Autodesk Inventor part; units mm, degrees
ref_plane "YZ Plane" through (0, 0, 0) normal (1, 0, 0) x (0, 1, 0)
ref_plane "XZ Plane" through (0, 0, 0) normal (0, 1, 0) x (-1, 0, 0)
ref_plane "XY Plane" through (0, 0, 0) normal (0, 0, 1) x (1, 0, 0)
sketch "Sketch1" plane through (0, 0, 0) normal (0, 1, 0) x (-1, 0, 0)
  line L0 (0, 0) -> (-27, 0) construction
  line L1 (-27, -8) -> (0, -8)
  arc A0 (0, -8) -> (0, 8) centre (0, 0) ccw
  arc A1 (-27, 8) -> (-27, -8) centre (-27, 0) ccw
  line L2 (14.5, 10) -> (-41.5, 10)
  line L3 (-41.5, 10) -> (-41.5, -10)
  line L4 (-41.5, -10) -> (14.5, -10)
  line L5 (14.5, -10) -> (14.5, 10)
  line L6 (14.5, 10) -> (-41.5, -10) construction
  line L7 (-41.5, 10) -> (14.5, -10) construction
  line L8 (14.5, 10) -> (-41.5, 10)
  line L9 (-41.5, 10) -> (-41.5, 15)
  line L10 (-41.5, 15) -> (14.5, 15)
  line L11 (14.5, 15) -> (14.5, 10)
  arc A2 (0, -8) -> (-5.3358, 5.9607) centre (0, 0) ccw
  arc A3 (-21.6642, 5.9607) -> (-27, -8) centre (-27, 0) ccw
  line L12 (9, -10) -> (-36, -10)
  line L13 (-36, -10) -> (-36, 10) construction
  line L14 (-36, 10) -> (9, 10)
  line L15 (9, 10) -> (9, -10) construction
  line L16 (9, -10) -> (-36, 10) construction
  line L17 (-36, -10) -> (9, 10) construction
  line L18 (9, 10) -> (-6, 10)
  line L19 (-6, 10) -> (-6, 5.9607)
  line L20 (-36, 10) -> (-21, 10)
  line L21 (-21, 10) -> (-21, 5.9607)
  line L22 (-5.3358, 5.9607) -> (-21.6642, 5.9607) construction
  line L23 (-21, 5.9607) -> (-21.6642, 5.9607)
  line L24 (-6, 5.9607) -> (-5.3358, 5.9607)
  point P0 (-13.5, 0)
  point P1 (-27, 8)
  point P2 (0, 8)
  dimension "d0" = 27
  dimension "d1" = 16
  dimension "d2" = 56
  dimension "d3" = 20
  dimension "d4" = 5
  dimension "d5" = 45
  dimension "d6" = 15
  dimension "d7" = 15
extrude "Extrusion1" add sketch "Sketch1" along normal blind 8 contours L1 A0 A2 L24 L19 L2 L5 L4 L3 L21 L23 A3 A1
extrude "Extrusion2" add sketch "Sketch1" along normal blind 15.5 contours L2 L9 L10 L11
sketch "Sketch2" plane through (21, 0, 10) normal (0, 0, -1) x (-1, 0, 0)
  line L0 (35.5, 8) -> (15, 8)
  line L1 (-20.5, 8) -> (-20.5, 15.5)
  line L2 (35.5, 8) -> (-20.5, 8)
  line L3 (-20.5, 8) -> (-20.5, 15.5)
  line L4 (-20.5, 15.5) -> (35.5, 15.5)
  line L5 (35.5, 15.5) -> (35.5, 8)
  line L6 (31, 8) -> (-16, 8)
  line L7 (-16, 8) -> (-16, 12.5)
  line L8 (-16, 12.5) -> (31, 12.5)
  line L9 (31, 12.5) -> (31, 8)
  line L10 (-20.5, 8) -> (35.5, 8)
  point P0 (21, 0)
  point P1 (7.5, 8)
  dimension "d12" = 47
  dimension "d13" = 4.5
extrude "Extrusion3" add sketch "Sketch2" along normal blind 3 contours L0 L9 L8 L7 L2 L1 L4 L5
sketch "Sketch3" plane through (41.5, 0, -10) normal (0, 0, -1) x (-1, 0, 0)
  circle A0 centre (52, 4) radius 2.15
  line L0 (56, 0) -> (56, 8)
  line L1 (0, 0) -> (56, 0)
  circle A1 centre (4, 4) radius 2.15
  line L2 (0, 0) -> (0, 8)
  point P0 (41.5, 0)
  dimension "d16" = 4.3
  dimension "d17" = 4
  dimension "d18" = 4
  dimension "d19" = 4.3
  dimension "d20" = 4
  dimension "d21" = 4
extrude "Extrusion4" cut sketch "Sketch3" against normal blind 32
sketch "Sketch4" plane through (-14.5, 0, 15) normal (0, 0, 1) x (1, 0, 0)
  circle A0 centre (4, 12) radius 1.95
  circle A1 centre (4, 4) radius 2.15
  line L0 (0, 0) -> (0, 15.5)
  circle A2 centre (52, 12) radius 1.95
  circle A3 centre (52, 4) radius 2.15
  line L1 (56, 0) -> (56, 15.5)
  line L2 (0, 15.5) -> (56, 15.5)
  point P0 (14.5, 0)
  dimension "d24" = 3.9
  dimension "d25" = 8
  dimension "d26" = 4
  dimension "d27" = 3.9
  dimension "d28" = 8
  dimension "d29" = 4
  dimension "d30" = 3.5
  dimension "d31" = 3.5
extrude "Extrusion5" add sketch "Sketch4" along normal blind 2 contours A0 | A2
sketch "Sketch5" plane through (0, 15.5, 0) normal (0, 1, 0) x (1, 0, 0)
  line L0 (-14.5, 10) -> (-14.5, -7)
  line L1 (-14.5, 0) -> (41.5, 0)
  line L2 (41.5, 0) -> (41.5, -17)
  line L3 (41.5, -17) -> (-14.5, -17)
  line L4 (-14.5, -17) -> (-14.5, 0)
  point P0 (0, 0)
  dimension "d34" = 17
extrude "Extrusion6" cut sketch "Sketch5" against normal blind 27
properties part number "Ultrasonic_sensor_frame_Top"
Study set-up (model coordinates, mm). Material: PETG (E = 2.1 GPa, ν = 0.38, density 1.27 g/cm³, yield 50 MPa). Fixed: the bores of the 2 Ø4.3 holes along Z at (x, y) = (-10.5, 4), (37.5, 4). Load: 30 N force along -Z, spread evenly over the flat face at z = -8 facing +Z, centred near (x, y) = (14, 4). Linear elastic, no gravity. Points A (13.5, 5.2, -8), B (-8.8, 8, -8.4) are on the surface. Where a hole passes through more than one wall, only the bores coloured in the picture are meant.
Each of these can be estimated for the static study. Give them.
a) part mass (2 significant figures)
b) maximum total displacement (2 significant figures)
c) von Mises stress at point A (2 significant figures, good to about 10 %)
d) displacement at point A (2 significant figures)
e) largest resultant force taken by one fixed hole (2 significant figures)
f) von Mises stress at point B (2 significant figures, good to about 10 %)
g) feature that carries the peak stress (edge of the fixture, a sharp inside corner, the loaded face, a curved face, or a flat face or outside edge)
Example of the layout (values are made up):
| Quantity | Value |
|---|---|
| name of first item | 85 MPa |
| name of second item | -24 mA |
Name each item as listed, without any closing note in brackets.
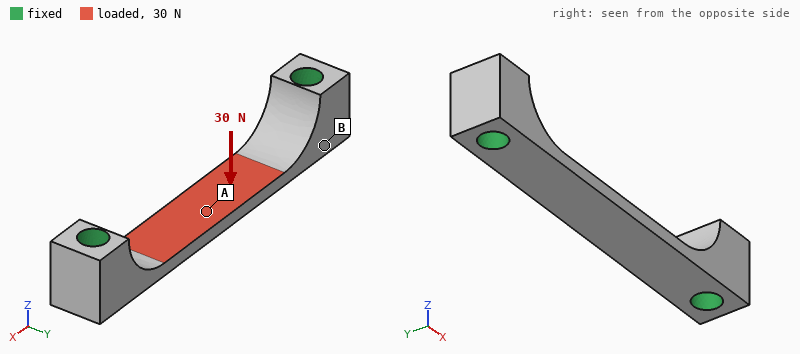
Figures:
| Quantity | Value |
|---|---|
| part mass | 2.1 g |
| maximum total displacement | 0.38 mm |
| von Mises stress at point A | 8.7 MPa |
| displacement at point A | 0.37 mm |
| largest resultant force taken by one fixed hole | 21 N |
| von Mises stress at point B | 1.6 MPa |
| feature that carries the peak stress | a curved face |
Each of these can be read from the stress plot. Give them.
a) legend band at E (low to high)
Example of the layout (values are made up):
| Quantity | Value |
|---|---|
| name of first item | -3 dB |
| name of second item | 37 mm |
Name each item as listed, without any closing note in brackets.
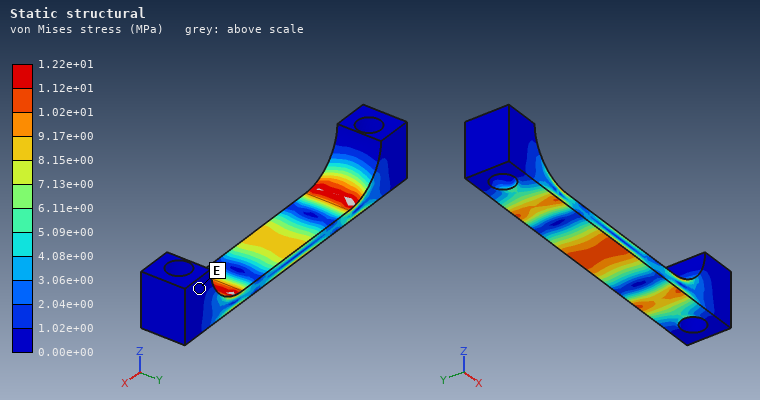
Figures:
| Quantity | Value |
|---|---|
| legend band at E | 0.00e+00 to 1.02e+00 MPa |
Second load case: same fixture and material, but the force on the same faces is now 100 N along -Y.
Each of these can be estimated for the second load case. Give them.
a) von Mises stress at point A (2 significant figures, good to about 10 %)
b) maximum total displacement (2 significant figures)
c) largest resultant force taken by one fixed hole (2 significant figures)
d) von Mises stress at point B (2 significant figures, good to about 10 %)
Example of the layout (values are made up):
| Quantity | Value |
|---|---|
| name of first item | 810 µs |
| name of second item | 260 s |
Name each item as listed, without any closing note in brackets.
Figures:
| Quantity | Value |
|---|---|
| von Mises stress at point A | 2.9 MPa |
| maximum total displacement | 0.30 mm |
| largest resultant force taken by one fixed hole | 50 N |
| von Mises stress at point B | 7.4 MPa |
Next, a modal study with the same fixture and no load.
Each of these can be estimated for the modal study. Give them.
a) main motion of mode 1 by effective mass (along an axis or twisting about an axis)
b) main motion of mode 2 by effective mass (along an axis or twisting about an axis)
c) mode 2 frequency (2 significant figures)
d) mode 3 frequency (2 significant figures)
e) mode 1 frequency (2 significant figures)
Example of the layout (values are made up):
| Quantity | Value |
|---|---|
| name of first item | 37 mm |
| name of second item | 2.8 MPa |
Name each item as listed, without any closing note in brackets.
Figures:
| Quantity | Value |
|---|---|
| main motion of mode 1 by effective mass | along Z |
| main motion of mode 2 by effective mass | along Y |
| mode 2 frequency | 4800 Hz |
| mode 3 frequency | 5400 Hz |
| mode 1 frequency | 2200 Hz |
